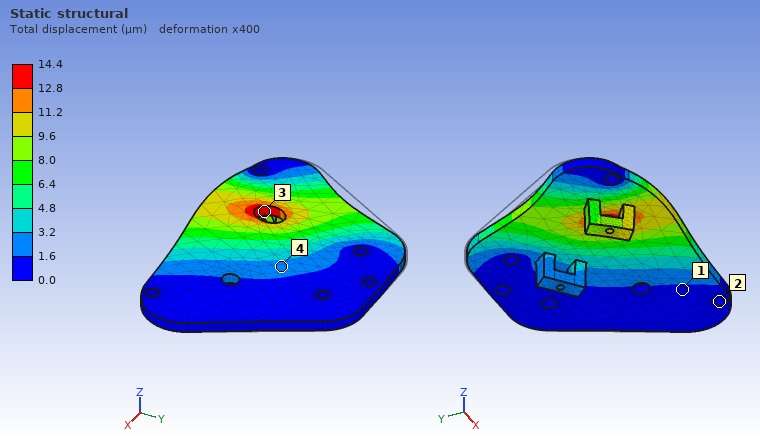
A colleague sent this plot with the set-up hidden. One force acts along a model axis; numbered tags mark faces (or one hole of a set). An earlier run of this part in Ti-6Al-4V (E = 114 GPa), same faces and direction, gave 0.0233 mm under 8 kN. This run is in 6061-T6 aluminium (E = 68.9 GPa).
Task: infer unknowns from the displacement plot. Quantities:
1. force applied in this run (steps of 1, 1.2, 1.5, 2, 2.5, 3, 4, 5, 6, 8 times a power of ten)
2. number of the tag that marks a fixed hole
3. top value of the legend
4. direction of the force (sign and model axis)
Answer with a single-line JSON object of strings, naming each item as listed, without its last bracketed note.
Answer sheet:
{"force applied in this run": "3 kN", "number of the tag that marks a fixed hole": "2", "top value of the legend": "14.4 µm", "direction of the force": "-Y"}
